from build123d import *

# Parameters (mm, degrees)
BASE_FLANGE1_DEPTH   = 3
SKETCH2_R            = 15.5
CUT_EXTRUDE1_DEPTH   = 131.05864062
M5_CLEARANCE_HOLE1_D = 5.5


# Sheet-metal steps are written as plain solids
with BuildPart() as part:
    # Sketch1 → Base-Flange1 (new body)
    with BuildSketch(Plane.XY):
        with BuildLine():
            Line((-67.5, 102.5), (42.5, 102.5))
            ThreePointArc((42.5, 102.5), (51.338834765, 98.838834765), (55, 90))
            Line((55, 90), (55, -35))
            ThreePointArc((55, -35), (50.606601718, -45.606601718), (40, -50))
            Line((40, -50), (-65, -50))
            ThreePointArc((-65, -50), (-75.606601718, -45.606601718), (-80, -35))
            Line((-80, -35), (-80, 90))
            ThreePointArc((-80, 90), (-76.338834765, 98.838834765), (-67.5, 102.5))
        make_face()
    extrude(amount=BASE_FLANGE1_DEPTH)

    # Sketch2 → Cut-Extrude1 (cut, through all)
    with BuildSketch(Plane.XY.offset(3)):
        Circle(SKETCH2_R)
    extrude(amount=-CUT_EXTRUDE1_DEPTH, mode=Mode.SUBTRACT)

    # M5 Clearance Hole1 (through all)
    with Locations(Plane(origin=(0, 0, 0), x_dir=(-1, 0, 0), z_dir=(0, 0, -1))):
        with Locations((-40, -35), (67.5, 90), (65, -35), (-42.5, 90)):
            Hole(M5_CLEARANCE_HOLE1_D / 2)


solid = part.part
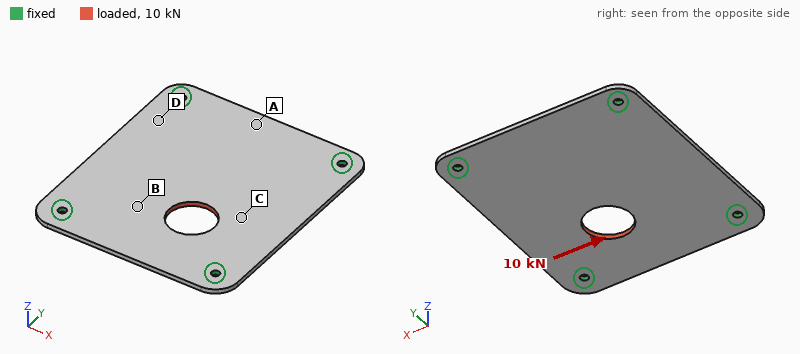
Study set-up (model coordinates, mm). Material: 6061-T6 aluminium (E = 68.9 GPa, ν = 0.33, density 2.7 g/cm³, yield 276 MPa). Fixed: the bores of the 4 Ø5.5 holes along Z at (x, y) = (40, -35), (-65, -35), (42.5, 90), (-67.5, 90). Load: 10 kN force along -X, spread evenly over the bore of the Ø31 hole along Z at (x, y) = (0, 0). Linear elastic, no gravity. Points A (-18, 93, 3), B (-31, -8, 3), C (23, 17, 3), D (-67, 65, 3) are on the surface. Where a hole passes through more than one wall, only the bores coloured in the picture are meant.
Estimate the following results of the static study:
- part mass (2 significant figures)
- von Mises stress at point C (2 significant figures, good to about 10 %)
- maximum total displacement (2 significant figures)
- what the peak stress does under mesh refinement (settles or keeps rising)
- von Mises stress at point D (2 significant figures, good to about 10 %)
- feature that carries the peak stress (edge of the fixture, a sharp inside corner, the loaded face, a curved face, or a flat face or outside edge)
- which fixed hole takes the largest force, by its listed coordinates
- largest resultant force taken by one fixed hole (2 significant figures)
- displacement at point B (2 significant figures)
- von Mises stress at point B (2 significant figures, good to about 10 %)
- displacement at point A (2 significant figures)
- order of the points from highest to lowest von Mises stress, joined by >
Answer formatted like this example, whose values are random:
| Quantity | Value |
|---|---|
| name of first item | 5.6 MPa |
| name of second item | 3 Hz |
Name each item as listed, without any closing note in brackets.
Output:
| Quantity | Value |
|---|---|
| part mass | 160 g |
| von Mises stress at point C | 23 MPa |
| maximum total displacement | 47 µm |
| what the peak stress does under mesh refinement | keeps rising |
| von Mises stress at point D | 12 MPa |
| feature that carries the peak stress | edge of the fixture |
| which fixed hole takes the largest force, by its listed coordinates | (40, -35) |
| largest resultant force taken by one fixed hole | 3.8 kN |
| displacement at point B | 27 µm |
| von Mises stress at point B | 31 MPa |
| displacement at point A | 7.9 µm |
| order of the points from highest to lowest von Mises stress, joined by > | B > C > D > A |
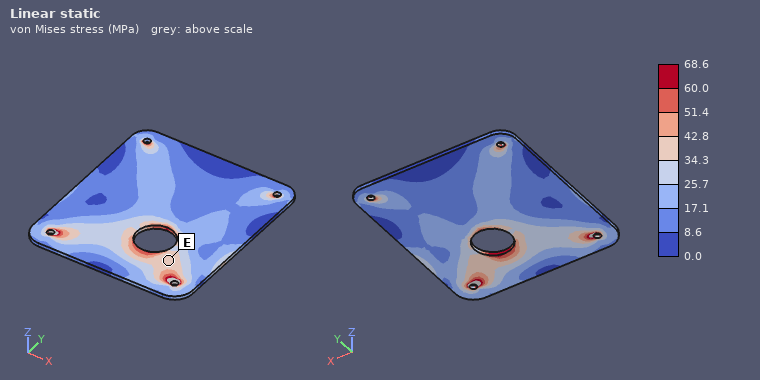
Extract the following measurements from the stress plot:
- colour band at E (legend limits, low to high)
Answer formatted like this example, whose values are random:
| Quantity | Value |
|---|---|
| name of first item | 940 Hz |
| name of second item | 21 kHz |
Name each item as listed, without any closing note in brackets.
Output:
| Quantity | Value |
|---|---|
| colour band at E | 34.3 to 42.8 MPa |
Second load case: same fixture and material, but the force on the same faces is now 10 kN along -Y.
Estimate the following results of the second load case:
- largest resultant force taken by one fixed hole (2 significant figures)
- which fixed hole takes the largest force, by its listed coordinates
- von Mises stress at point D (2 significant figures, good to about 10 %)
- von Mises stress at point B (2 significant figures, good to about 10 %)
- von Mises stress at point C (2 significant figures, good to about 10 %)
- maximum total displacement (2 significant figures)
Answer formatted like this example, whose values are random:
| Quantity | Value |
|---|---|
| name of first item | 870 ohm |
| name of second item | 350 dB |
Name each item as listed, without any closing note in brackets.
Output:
| Quantity | Value |
|---|---|
| largest resultant force taken by one fixed hole | 3.7 kN |
| which fixed hole takes the largest force, by its listed coordinates | (40, -35) |
| von Mises stress at point D | 16 MPa |
| von Mises stress at point B | 22 MPa |
| von Mises stress at point C | 30 MPa |
| maximum total displacement | 48 µm |
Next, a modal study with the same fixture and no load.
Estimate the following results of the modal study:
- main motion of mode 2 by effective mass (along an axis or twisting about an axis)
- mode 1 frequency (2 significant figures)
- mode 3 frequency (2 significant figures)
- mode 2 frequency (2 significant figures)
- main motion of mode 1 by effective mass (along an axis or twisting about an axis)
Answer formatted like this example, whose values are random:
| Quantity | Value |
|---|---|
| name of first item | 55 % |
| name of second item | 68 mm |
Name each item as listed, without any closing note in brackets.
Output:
| Quantity | Value |
|---|---|
| main motion of mode 2 by effective mass | twisting about Y |
| mode 1 frequency | 760 Hz |
| mode 3 frequency | 1400 Hz |
| mode 2 frequency | 1100 Hz |
| main motion of mode 1 by effective mass | along Z |
